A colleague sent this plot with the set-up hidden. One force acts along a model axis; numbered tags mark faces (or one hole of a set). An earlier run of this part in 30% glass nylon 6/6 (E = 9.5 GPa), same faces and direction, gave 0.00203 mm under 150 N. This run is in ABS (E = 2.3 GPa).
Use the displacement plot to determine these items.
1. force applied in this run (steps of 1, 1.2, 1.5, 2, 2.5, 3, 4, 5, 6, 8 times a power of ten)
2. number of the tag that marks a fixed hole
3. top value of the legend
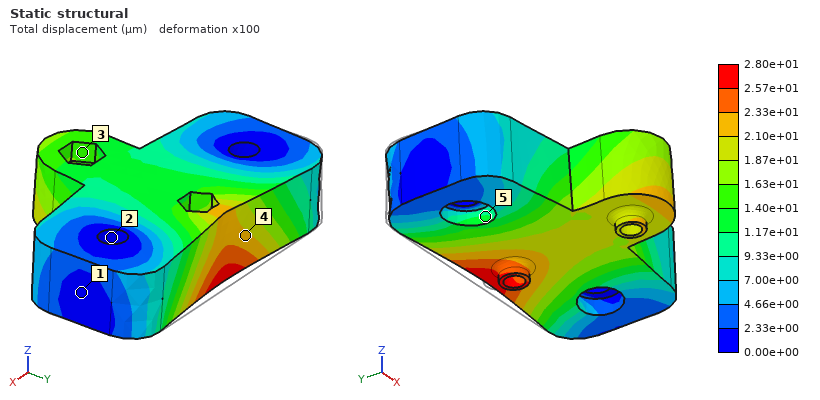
500 N
2
2.80e+01 µm
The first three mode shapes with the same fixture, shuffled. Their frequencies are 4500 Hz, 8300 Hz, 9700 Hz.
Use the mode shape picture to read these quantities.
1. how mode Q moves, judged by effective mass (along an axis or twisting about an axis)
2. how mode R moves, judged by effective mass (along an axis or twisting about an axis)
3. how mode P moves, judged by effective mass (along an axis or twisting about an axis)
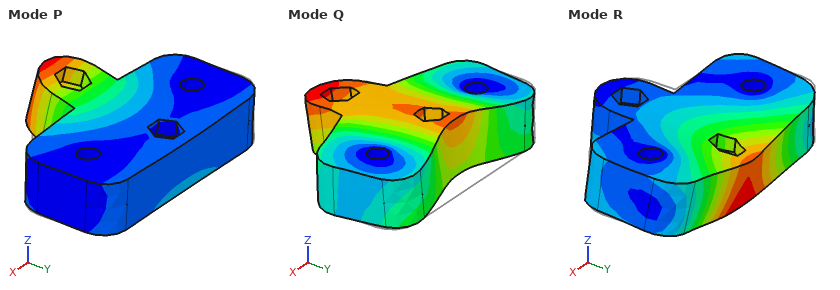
along Y
along Z
along Z
